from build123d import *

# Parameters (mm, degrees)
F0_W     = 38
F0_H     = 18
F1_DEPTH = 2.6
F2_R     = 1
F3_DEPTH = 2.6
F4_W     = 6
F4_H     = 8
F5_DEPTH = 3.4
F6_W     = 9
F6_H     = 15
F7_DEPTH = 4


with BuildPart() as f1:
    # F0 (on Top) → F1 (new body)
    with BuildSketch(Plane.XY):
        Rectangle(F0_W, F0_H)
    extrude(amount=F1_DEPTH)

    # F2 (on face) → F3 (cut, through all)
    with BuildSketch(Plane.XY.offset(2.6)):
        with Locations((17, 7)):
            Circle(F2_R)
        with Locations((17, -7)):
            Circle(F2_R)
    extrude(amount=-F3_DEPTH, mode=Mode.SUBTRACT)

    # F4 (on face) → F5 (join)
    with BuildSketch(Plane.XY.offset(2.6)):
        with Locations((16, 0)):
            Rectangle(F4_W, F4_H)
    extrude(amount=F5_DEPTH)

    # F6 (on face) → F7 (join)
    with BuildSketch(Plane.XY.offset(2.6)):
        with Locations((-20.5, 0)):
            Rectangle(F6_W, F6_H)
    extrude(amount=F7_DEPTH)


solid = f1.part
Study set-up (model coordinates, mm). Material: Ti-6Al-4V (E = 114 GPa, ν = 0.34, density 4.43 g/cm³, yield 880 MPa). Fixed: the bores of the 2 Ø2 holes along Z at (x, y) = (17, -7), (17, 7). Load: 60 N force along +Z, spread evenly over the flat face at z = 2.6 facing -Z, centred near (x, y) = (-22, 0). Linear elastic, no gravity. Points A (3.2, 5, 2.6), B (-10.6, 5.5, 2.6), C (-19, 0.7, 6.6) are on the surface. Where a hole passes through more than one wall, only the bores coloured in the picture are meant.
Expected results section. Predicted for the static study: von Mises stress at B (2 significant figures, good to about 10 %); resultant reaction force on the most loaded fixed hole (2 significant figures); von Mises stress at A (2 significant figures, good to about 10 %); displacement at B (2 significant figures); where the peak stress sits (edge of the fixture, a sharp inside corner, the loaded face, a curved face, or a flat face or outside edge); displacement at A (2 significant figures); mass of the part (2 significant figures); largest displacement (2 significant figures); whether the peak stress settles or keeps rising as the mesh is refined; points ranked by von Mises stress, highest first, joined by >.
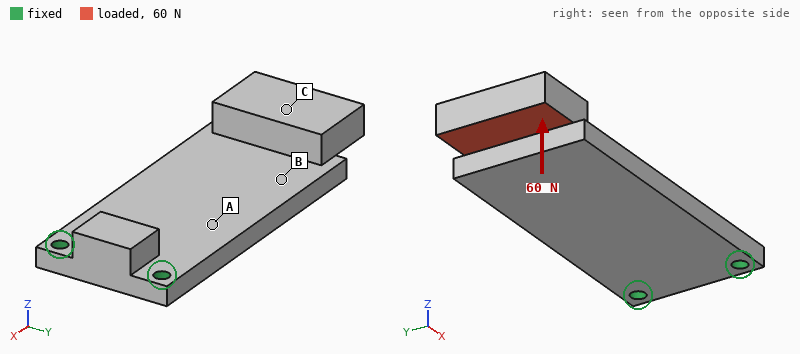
34 MPa
32 N
74 MPa
0.23 mm
edge of the fixture
0.070 mm
11 g
0.45 mm
keeps rising
A > B > C
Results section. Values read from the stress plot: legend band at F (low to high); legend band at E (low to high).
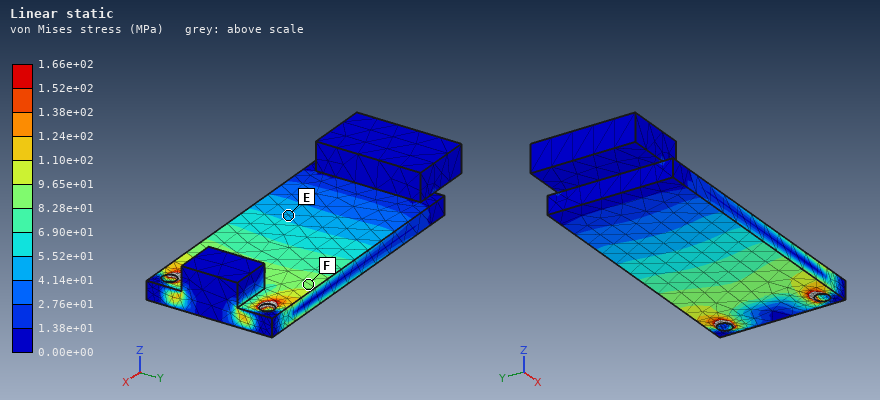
8.28e+01 to 9.65e+01 MPa
4.14e+01 to 5.52e+01 MPa
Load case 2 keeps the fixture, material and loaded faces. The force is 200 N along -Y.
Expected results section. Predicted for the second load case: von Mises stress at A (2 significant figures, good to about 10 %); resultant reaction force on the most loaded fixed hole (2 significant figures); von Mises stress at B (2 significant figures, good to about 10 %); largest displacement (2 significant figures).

27 MPa
550 N
21 MPa
45 µm
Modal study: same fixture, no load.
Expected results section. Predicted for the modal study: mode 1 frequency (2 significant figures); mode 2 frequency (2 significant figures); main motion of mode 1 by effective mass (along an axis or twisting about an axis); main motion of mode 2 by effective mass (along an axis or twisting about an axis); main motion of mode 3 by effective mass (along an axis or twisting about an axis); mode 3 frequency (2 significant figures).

1000 Hz
4800 Hz
along Z
along Y
along Z
6700 Hz
